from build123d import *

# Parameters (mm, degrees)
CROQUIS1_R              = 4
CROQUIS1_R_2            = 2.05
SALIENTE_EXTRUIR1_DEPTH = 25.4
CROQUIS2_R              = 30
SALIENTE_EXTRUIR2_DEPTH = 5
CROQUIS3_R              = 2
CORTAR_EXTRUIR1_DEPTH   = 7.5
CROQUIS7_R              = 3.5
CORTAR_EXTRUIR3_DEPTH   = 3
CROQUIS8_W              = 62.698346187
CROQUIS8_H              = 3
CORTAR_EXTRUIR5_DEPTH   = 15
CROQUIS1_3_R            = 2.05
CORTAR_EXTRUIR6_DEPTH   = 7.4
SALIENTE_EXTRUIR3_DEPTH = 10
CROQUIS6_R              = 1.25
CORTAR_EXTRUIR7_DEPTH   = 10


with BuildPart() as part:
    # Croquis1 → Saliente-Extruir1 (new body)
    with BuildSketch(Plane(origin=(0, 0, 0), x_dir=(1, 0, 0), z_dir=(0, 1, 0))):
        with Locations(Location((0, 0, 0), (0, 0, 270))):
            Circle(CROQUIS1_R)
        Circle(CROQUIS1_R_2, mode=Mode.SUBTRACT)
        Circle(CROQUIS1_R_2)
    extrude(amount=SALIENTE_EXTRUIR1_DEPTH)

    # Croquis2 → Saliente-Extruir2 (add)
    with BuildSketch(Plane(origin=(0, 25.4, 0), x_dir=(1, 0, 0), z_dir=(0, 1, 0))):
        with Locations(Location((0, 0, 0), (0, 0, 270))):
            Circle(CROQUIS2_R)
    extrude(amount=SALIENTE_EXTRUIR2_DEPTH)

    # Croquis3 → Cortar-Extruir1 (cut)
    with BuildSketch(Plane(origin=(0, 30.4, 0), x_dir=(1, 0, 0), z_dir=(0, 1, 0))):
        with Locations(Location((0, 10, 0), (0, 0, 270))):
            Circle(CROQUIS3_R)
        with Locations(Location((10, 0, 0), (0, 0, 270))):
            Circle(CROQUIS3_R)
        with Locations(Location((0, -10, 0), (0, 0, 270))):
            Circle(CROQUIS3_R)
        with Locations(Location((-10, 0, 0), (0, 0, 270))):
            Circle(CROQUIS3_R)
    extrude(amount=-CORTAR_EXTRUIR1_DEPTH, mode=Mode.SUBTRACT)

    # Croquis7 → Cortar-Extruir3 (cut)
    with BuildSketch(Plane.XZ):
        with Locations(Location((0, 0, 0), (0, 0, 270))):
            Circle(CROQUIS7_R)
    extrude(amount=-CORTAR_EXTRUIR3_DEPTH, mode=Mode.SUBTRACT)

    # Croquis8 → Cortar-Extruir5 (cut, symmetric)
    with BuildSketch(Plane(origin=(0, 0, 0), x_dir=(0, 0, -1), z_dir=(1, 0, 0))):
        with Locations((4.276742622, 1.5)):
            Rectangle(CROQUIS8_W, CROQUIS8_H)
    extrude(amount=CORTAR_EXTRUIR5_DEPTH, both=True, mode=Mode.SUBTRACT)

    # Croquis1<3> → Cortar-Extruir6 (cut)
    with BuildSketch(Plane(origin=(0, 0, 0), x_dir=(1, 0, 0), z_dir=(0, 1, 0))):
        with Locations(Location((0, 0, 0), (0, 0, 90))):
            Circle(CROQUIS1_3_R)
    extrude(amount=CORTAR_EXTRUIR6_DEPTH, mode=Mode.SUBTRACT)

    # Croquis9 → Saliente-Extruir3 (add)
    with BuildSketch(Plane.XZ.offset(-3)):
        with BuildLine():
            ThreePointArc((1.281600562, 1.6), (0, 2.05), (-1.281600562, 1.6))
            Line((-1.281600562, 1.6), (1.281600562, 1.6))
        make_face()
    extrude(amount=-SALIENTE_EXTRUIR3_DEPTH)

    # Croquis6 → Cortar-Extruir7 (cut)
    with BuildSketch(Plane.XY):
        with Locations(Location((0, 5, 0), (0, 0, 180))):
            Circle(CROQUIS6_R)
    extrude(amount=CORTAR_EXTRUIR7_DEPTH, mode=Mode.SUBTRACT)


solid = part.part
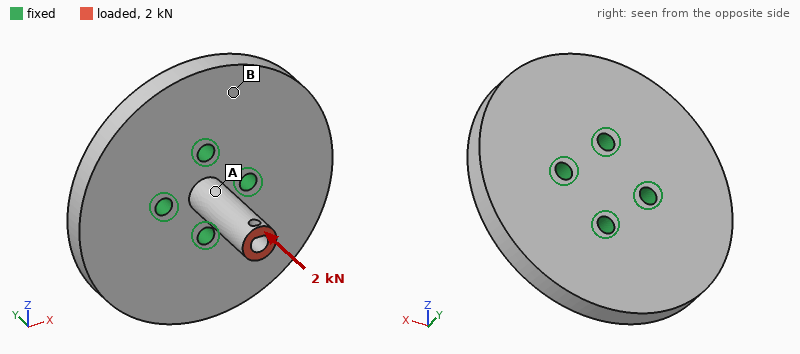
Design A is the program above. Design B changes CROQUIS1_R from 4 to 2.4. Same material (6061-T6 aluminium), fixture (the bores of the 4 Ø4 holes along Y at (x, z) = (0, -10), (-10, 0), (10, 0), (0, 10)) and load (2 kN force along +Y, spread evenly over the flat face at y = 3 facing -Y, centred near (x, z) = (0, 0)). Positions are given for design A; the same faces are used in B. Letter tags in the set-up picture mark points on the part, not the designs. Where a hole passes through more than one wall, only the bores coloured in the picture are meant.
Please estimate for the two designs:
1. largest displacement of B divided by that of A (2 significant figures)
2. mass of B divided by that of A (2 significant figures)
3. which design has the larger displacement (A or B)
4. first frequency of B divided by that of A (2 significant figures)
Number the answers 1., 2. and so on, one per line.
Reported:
1. 8.5
2. 0.95
3. B
4. 0.87
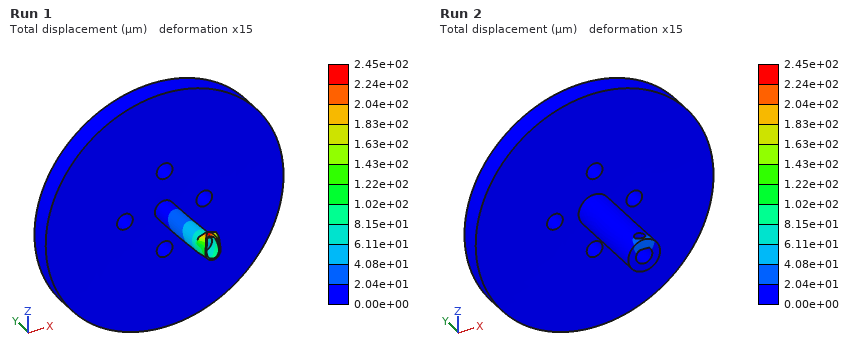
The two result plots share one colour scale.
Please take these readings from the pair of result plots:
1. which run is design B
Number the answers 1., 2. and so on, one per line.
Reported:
1. Run 1
